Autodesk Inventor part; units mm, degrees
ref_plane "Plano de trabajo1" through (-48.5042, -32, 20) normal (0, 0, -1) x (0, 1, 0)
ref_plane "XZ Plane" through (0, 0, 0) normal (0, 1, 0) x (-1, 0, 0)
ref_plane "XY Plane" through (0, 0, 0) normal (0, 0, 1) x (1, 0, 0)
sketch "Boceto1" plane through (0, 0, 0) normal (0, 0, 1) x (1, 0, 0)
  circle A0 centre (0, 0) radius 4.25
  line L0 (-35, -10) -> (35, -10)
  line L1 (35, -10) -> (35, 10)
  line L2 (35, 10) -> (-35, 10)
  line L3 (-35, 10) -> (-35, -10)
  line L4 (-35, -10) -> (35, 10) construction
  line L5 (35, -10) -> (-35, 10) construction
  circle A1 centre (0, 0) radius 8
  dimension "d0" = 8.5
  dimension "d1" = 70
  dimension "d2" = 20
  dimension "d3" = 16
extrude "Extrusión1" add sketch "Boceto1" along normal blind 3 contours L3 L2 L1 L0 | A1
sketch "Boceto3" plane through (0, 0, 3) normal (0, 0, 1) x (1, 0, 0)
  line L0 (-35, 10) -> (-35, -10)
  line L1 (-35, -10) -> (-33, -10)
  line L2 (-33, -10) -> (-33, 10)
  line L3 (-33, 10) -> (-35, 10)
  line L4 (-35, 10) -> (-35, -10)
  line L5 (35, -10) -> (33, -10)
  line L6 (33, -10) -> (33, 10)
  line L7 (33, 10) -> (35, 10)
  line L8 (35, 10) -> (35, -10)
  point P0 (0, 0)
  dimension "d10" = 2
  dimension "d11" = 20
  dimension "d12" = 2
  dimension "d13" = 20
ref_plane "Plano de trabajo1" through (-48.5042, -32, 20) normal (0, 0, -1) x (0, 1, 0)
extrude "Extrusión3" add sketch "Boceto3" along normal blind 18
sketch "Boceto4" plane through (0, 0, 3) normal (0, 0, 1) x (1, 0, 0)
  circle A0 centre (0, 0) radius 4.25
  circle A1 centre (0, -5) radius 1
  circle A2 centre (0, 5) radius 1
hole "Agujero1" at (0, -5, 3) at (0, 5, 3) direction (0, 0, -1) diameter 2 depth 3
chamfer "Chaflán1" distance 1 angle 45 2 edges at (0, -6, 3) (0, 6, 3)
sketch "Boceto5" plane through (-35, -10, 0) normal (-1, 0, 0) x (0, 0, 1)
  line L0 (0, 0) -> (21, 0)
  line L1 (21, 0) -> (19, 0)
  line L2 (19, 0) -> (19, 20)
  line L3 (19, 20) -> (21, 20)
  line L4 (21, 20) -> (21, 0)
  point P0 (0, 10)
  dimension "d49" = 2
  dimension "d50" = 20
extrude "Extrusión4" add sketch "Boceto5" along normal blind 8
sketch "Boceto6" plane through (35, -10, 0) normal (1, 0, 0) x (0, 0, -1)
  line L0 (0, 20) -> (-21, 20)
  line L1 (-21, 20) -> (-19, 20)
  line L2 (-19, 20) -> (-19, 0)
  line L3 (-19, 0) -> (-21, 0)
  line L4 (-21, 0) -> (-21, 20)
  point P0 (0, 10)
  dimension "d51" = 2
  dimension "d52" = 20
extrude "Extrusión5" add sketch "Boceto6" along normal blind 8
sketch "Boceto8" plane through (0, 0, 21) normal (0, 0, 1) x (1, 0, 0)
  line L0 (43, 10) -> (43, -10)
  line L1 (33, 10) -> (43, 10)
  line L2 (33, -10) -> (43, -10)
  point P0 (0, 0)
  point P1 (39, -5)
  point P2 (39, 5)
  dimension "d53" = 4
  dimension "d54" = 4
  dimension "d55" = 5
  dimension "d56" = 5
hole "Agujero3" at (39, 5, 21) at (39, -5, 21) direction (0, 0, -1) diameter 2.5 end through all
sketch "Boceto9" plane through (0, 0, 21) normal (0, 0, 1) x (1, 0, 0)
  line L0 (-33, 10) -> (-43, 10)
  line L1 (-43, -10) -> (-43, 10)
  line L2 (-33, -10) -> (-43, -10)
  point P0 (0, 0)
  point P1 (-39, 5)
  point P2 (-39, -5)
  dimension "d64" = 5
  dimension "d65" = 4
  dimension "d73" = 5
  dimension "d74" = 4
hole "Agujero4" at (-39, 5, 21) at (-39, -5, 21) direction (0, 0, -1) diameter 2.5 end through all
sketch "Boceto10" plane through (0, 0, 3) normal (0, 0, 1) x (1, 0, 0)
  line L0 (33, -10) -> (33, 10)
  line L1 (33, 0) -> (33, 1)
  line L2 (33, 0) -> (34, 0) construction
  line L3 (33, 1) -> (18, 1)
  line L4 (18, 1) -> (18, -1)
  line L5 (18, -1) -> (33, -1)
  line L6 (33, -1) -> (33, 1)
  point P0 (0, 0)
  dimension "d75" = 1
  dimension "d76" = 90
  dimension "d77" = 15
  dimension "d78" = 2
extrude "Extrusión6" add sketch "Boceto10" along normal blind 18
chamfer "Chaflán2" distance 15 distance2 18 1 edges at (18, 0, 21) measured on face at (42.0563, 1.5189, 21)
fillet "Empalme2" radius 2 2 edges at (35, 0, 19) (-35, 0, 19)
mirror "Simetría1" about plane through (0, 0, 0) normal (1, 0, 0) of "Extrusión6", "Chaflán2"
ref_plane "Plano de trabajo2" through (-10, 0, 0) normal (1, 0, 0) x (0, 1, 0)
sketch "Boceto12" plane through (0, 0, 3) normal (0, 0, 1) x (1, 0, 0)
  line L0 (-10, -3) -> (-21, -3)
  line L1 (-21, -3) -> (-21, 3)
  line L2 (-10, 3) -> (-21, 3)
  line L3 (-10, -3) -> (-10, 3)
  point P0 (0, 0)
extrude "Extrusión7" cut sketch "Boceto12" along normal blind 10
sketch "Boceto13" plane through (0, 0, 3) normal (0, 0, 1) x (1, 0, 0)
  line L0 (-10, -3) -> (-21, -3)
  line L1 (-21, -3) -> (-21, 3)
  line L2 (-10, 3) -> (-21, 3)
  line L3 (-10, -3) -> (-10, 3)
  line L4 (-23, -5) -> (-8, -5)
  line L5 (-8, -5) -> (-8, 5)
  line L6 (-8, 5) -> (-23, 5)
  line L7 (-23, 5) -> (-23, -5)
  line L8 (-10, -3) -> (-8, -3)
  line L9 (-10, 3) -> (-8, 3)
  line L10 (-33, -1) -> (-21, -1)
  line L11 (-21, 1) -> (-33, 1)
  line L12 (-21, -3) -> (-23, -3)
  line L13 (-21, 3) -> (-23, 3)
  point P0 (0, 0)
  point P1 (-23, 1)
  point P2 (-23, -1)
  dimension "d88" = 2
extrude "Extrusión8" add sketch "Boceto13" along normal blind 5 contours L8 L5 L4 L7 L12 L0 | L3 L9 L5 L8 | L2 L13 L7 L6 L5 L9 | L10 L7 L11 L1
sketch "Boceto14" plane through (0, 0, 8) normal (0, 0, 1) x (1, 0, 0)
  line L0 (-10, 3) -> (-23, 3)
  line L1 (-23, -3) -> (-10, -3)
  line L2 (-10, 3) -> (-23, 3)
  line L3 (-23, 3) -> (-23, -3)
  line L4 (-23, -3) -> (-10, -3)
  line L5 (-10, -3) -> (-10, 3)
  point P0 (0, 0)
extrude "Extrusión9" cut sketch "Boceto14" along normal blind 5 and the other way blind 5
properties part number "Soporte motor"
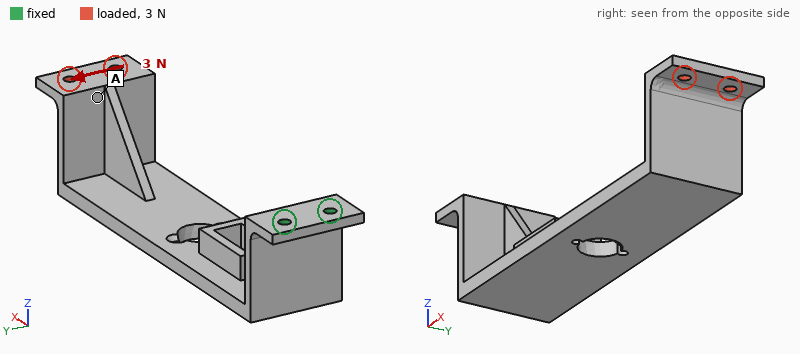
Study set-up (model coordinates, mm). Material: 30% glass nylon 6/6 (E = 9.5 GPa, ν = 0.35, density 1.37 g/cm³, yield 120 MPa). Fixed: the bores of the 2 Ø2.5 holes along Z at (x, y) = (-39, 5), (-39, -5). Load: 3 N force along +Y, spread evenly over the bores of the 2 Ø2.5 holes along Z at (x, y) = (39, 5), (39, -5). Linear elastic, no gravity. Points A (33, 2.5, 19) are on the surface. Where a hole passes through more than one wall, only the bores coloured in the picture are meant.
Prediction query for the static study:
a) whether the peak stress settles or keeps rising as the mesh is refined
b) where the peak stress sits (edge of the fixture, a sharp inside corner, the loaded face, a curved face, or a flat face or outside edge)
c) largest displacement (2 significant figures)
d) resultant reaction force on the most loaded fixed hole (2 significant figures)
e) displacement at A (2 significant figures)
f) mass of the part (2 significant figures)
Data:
keeps rising
edge of the fixture
0.89 mm
20 N
0.76 mm
9.5 g
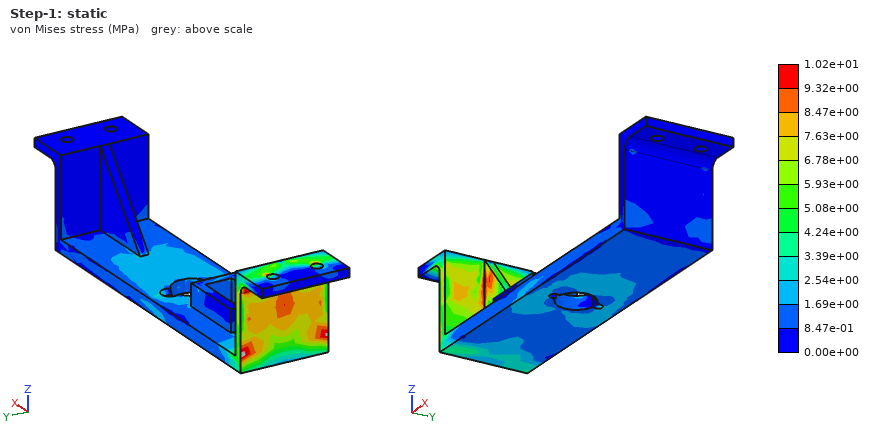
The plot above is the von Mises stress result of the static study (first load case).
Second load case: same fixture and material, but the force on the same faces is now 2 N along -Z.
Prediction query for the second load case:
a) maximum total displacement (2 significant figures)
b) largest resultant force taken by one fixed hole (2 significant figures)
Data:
1.0 mm
1.7 N
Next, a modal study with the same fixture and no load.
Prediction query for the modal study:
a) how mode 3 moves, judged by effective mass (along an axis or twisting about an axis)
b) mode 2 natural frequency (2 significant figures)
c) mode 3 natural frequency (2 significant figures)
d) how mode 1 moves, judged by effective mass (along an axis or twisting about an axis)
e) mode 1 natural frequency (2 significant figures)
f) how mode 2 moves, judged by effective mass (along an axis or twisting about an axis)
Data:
along X
180 Hz
540 Hz
along Z
140 Hz
along Y
